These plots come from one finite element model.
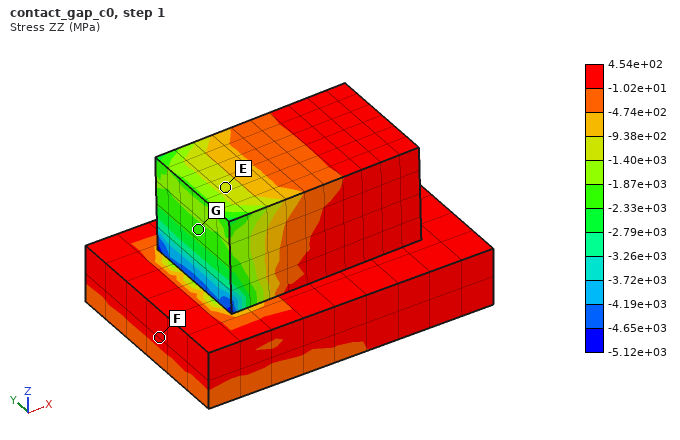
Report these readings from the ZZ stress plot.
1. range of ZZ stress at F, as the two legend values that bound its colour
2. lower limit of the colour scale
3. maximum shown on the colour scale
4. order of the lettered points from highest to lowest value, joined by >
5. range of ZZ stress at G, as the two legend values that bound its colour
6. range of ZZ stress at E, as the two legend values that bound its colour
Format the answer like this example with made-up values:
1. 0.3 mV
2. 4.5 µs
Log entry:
1. -1.02e+01 to 4.54e+02 MPa
2. -5.12e+03 MPa
3. 4.54e+02 MPa
4. F > E > G
5. -2.33e+03 to -1.87e+03 MPa
6. -1.40e+03 to -9.38e+02 MPa
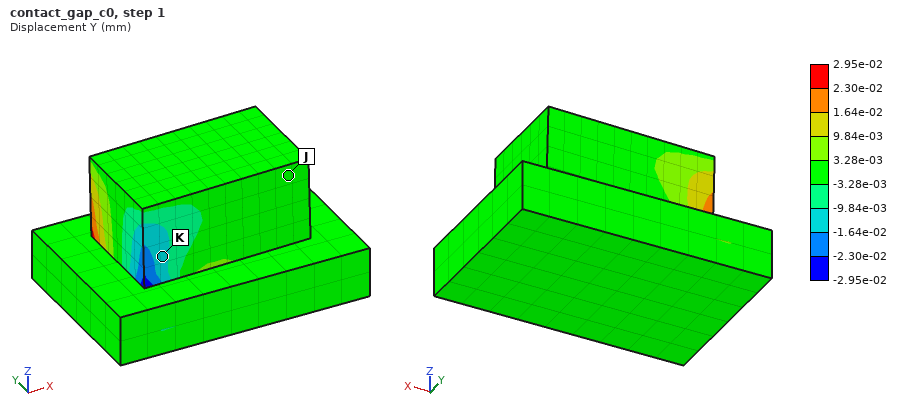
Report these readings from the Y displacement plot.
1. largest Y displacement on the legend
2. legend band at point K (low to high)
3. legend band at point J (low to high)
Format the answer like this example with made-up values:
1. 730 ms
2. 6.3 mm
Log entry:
1. 2.95e-02 mm
2. -1.64e-02 to -9.84e-03 mm
3. -3.28e-03 to 3.28e-03 mm
